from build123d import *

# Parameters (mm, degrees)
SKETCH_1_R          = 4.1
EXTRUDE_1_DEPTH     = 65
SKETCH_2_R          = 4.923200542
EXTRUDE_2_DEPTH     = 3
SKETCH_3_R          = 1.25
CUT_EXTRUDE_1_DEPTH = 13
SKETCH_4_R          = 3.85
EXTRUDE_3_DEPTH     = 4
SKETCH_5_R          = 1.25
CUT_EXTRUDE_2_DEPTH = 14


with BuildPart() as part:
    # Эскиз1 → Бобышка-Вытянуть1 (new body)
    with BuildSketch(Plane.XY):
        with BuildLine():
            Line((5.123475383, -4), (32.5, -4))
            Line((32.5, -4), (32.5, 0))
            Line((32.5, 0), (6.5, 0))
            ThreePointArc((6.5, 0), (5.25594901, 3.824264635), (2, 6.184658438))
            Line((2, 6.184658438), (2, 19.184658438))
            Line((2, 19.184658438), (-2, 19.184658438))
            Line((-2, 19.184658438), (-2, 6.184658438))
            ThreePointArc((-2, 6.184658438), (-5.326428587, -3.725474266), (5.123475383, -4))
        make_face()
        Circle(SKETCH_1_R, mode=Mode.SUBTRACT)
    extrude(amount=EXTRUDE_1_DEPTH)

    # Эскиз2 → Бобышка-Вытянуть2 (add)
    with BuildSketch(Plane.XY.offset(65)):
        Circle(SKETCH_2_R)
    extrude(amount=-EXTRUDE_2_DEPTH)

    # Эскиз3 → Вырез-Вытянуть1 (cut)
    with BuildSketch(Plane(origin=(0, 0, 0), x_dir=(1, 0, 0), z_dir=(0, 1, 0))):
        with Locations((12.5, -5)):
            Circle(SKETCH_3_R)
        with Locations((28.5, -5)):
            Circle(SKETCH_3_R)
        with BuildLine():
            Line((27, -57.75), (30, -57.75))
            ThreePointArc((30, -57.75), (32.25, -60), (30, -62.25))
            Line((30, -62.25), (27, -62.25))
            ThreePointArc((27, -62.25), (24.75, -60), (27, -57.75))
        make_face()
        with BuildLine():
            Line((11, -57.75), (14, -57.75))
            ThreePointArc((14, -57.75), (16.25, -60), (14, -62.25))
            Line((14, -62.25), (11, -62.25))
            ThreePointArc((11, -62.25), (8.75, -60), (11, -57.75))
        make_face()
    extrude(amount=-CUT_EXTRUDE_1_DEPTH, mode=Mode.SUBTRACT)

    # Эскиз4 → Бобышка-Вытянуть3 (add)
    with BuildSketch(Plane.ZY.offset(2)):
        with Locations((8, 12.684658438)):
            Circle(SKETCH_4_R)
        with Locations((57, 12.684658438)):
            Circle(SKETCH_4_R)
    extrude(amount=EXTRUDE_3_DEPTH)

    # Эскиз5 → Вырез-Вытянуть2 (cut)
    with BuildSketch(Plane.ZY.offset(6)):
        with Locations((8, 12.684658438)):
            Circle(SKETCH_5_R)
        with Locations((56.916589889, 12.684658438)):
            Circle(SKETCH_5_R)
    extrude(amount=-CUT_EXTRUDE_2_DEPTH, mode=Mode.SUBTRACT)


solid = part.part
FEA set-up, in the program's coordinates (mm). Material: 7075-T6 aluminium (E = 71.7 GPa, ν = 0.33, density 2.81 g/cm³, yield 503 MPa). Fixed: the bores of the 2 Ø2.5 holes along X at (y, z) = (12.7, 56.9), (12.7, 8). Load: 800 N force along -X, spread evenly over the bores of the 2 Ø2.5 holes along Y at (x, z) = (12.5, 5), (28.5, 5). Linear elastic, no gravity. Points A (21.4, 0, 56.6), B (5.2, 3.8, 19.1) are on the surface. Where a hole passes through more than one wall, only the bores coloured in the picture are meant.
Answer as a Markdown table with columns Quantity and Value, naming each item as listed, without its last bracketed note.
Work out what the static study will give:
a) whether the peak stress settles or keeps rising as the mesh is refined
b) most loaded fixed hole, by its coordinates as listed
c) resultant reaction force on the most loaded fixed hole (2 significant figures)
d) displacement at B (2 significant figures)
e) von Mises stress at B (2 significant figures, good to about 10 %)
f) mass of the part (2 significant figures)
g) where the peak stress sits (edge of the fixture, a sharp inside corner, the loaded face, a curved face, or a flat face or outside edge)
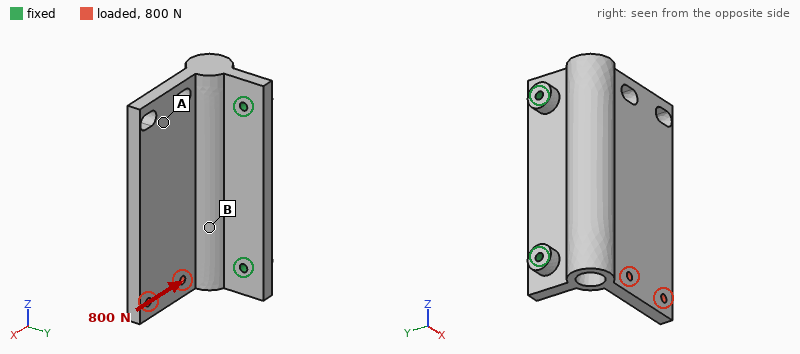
| Quantity | Value |
|---|---|
| whether the peak stress settles or keeps rising as the mesh is refined | keeps rising |
| most loaded fixed hole, by its coordinates as listed | (12.7, 8) |
| resultant reaction force on the most loaded fixed hole | 830 N |
| displacement at B | 0.041 mm |
| von Mises stress at B | 27 MPa |
| mass of the part | 44 g |
| where the peak stress sits | edge of the fixture |
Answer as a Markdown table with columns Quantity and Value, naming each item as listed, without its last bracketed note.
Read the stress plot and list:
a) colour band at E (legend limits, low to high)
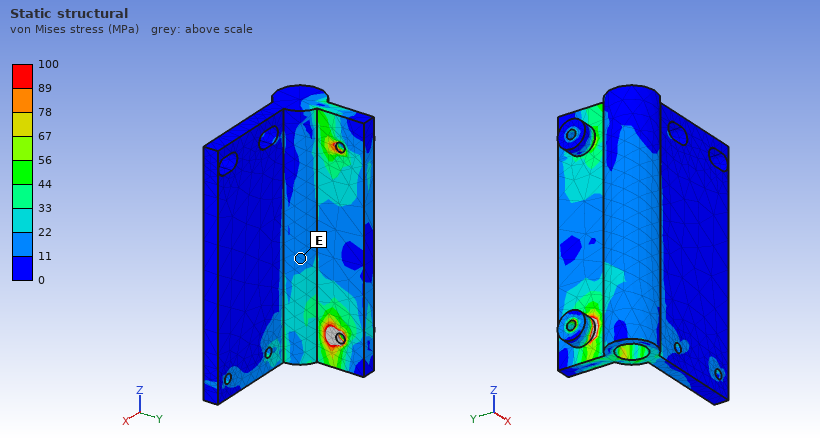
| Quantity | Value |
|---|---|
| colour band at E | 11 to 22 MPa |
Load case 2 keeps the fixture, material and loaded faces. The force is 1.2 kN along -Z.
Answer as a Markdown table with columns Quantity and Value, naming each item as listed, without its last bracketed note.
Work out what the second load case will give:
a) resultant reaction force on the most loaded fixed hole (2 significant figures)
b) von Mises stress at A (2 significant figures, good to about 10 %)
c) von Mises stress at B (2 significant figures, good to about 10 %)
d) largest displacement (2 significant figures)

| Quantity | Value |
|---|---|
| resultant reaction force on the most loaded fixed hole | 850 N |
| von Mises stress at A | 6.2 MPa |
| von Mises stress at B | 26 MPa |
| largest displacement | 49 µm |
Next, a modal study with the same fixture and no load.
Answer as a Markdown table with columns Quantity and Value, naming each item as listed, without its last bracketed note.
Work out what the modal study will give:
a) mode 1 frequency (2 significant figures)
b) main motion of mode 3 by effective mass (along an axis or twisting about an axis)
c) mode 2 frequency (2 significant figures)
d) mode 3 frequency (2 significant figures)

| Quantity | Value |
|---|---|
| mode 1 frequency | 1800 Hz |
| main motion of mode 3 by effective mass | along X |
| mode 2 frequency | 4700 Hz |
| mode 3 frequency | 6200 Hz |
